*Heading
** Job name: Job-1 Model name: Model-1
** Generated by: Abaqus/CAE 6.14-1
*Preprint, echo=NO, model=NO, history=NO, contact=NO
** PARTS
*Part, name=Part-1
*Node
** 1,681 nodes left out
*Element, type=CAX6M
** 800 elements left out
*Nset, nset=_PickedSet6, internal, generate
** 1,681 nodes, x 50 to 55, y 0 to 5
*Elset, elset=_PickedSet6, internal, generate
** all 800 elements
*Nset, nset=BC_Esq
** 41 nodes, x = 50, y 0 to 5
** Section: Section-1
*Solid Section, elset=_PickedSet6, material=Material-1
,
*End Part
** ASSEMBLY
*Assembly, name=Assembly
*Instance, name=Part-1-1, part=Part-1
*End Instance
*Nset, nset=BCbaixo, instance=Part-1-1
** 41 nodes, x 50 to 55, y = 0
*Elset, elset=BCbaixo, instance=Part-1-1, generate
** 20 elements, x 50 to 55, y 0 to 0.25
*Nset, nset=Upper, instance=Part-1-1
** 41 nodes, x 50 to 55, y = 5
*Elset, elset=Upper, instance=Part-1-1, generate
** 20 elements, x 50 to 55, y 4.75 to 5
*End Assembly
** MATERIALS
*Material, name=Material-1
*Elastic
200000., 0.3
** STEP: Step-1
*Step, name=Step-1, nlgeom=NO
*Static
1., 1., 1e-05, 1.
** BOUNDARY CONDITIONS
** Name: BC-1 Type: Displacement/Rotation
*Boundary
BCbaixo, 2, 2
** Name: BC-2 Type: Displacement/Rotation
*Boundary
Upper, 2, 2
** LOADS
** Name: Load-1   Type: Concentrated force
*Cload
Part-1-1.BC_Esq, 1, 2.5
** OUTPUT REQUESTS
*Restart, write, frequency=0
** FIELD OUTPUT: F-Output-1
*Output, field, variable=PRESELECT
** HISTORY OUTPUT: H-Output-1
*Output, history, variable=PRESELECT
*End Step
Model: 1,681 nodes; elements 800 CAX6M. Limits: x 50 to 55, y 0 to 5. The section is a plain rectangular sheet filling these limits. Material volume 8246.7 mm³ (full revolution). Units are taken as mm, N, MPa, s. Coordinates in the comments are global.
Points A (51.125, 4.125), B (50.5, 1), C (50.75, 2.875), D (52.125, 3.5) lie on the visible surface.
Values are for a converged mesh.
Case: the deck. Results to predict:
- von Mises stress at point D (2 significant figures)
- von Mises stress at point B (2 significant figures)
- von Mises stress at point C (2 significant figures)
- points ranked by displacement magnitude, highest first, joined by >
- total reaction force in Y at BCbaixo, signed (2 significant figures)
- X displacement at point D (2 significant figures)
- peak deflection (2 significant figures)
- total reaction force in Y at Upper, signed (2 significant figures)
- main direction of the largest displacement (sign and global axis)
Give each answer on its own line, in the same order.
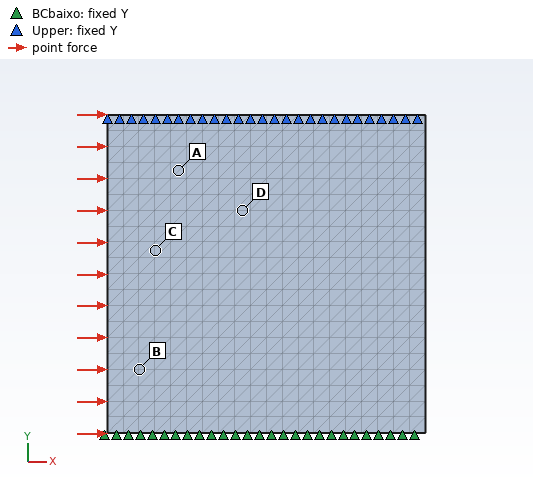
0.61 MPa
0.65 MPa
0.64 MPa
B > C > A > D
-310 N
1.6e-04 mm
1.6e-04 mm
310 N
+X
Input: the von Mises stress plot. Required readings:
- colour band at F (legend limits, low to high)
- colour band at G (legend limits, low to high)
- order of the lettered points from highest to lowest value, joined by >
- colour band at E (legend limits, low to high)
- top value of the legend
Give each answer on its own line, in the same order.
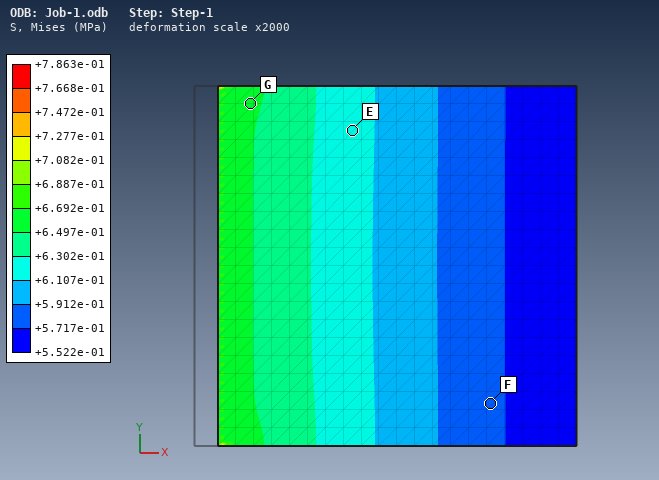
+5.717e-01 to +5.912e-01 MPa
+6.497e-01 to +6.692e-01 MPa
G > E > F
+6.107e-01 to +6.302e-01 MPa
+7.863e-01 MPa
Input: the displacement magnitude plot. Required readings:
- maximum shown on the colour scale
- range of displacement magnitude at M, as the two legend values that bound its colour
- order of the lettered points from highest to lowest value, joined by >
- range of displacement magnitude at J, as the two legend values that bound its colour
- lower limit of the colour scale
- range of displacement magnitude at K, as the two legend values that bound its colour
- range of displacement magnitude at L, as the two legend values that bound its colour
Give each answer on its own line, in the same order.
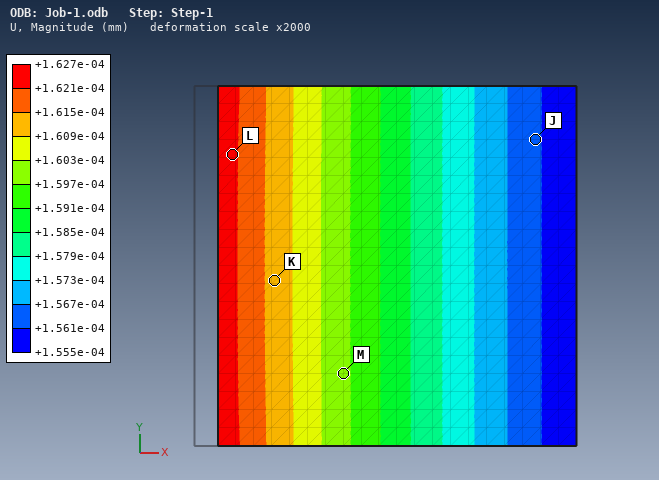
+1.627e-04 mm
+1.597e-04 to +1.603e-04 mm
L > K > M > J
+1.561e-04 to +1.567e-04 mm
+1.555e-04 mm
+1.609e-04 to +1.615e-04 mm
+1.621e-04 to +1.627e-04 mm
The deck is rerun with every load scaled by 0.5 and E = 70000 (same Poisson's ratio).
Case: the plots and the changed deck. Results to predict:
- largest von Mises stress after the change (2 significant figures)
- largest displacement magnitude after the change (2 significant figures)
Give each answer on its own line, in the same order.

0.39 MPa
2.3e-04 mm
